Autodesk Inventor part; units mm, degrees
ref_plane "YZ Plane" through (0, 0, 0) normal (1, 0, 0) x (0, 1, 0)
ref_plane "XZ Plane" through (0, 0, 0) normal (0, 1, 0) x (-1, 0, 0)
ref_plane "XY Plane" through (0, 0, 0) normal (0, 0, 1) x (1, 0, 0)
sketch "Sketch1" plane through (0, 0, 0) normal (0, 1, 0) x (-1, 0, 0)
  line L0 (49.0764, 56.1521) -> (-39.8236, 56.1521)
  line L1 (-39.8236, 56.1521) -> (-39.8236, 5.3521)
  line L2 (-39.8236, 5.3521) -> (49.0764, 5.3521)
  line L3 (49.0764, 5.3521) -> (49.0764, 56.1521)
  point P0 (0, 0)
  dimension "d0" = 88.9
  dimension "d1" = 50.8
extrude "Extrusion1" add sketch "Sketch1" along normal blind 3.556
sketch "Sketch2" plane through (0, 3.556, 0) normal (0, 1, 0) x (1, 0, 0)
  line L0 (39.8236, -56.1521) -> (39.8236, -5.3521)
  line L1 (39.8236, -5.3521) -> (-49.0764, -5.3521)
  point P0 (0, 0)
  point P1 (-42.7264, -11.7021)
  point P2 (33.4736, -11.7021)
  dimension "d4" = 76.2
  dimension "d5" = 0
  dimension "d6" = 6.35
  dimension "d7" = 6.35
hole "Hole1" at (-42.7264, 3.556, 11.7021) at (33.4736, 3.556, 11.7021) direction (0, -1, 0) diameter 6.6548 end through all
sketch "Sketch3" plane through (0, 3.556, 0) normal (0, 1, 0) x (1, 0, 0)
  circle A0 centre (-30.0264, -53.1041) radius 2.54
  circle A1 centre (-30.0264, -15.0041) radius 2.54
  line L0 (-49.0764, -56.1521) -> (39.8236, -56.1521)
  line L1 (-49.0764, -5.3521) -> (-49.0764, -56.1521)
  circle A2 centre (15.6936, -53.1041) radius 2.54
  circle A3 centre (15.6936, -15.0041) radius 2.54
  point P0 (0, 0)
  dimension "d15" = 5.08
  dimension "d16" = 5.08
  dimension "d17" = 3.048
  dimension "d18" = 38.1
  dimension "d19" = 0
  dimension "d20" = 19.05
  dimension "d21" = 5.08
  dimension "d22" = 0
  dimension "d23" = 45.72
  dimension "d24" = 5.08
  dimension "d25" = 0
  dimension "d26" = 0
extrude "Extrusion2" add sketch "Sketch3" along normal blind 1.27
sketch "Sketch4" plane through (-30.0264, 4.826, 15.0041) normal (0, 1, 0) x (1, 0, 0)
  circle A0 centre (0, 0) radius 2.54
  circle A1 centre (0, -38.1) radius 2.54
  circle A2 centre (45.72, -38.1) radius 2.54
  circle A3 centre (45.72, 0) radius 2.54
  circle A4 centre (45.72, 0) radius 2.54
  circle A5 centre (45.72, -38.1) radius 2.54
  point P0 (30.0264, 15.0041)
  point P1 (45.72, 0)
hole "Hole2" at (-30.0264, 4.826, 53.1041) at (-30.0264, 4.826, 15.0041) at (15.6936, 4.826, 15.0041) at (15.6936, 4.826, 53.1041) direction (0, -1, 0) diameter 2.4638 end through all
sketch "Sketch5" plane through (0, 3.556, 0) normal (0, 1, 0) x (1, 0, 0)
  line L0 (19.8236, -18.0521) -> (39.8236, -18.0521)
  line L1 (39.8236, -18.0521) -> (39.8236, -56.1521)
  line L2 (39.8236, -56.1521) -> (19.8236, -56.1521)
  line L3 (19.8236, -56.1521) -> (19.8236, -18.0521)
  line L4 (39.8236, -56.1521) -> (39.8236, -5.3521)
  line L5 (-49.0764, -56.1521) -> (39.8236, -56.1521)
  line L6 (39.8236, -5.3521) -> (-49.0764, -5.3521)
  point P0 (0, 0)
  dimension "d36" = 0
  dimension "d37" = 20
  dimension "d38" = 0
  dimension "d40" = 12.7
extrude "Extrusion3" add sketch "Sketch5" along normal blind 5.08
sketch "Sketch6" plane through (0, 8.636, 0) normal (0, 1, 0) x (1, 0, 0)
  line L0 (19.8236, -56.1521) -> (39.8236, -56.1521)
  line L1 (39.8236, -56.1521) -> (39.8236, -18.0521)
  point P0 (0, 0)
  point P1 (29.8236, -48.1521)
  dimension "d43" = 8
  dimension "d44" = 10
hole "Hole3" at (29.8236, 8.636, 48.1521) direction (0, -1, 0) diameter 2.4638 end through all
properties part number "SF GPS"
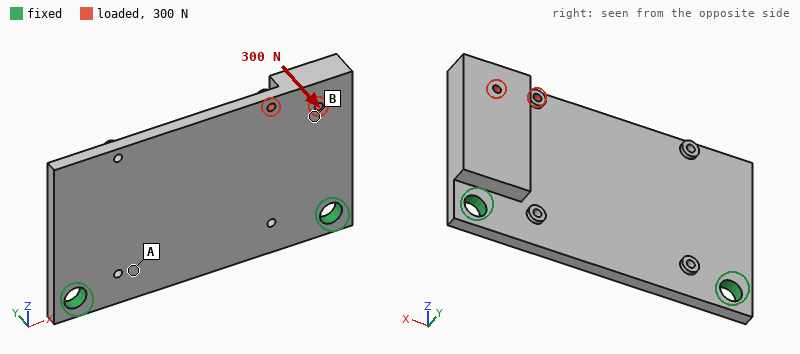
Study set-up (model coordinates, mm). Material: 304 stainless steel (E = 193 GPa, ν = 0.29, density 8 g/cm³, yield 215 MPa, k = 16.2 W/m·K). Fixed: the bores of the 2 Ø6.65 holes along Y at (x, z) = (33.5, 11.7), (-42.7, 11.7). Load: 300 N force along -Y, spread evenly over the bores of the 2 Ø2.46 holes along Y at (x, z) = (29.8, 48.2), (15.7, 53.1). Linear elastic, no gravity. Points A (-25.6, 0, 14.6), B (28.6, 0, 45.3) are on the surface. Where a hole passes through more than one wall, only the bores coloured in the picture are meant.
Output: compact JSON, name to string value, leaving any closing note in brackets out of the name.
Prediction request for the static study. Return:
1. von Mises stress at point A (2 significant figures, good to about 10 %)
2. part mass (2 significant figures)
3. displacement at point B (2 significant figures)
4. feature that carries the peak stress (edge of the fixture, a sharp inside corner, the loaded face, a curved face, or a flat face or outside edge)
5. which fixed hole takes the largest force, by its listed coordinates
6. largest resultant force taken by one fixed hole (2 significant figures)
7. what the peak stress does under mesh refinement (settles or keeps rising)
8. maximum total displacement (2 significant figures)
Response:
{"von Mises stress at point A": "30 MPa", "part mass": "160 g", "displacement at point B": "0.097 mm", "feature that carries the peak stress": "edge of the fixture", "which fixed hole takes the largest force, by its listed coordinates": "(33.5, 11.7)", "largest resultant force taken by one fixed hole": "270 N", "what the peak stress does under mesh refinement": "keeps rising", "maximum total displacement": "0.14 mm"}
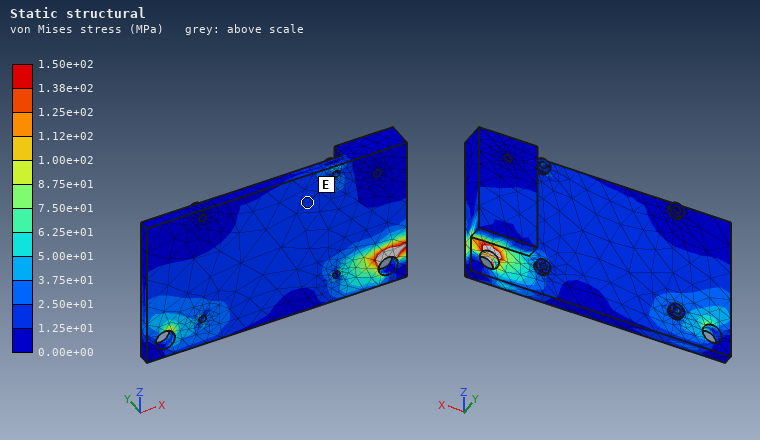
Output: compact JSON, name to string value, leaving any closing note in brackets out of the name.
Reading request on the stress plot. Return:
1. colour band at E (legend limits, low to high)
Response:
{"colour band at E": "1.25e+01 to 2.50e+01 MPa"}
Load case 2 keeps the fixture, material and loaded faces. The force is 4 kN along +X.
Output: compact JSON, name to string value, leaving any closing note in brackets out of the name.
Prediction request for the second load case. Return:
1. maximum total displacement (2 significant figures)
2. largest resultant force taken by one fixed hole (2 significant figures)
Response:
{"maximum total displacement": "30 µm", "largest resultant force taken by one fixed hole": "2.9 kN"}
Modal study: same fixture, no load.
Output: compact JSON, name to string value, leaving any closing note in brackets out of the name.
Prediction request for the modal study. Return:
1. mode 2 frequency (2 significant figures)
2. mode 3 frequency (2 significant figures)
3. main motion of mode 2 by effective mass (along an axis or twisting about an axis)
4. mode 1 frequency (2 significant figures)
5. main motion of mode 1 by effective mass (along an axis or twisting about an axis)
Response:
{"mode 2 frequency": "2200 Hz", "mode 3 frequency": "3300 Hz", "main motion of mode 2 by effective mass": "twisting about Z", "mode 1 frequency": "1100 Hz", "main motion of mode 1 by effective mass": "along Y"}
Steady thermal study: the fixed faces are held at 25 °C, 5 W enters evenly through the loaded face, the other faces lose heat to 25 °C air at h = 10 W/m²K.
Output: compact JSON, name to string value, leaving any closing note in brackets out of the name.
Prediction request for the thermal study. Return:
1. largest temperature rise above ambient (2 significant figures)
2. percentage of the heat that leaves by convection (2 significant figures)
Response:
{"largest temperature rise above ambient": "52 K", "percentage of the heat that leaves by convection": "36 %"}
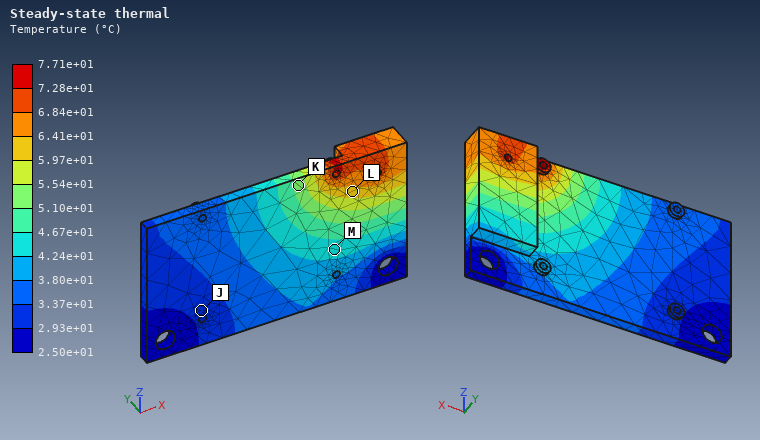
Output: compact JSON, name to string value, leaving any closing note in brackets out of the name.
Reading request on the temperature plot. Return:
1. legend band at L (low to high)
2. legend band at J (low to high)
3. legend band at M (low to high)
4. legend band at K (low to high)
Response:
{"legend band at L": "5.97e+01 to 6.41e+01 °C", "legend band at J": "2.93e+01 to 3.37e+01 °C", "legend band at M": "4.24e+01 to 4.67e+01 °C", "legend band at K": "5.10e+01 to 5.54e+01 °C"}
